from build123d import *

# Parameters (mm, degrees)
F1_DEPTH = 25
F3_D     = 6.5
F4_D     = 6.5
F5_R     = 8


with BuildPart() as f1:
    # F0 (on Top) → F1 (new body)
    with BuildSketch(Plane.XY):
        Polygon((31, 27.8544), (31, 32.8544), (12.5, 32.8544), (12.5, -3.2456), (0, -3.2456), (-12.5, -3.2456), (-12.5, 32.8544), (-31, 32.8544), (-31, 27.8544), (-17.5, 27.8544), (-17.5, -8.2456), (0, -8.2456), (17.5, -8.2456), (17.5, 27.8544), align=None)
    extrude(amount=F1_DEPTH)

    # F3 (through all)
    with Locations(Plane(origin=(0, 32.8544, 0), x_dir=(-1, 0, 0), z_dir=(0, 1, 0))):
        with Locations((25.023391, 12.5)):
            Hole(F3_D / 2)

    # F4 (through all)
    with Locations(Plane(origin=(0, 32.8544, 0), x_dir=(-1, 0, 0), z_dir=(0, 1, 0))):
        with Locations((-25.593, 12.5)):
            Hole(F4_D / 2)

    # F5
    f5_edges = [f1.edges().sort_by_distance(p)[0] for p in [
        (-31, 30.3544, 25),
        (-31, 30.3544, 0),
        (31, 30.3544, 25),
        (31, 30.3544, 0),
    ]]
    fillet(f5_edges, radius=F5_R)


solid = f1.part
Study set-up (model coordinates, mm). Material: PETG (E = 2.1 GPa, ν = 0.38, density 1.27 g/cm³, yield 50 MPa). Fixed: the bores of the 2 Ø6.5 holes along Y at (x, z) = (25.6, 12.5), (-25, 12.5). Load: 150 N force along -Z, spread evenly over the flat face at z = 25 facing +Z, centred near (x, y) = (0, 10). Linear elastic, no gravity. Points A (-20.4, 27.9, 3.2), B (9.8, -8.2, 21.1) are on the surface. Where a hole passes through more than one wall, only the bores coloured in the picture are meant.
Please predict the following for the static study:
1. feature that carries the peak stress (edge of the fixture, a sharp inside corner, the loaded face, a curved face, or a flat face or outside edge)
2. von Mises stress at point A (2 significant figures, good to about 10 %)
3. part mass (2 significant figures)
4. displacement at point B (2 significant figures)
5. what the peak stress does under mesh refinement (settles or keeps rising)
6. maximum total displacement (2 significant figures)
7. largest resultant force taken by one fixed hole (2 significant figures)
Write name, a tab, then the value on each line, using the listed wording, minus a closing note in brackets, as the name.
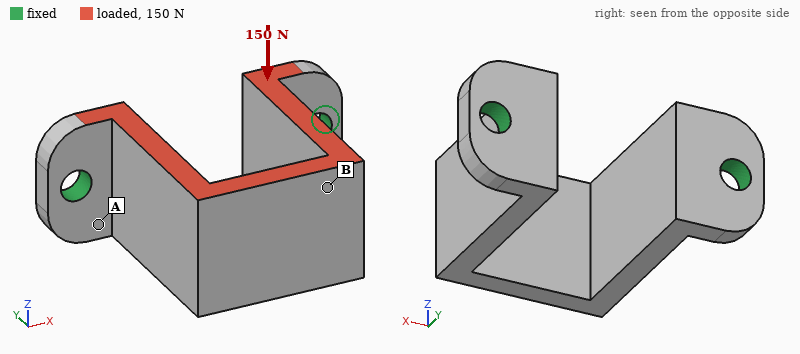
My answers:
feature that carries the peak stress	edge of the fixture
von Mises stress at point A	5.4 MPa
part mass	21 g
displacement at point B	0.60 mm
what the peak stress does under mesh refinement	keeps rising
maximum total displacement	0.62 mm
largest resultant force taken by one fixed hole	76 N
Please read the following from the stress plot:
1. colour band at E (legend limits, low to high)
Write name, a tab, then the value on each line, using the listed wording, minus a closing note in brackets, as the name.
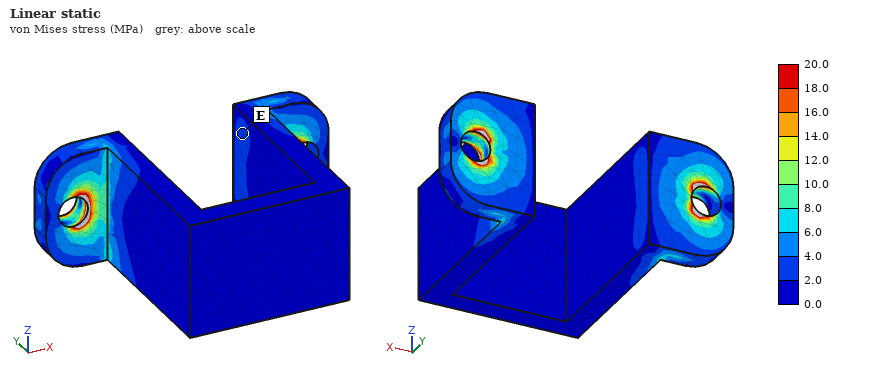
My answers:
colour band at E	2.0 to 4.0 MPa
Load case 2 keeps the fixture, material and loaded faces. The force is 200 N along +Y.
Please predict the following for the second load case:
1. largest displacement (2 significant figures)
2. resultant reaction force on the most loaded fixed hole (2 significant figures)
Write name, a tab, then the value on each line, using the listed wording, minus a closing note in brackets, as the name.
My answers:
largest displacement	0.51 mm
resultant reaction force on the most loaded fixed hole	100 N
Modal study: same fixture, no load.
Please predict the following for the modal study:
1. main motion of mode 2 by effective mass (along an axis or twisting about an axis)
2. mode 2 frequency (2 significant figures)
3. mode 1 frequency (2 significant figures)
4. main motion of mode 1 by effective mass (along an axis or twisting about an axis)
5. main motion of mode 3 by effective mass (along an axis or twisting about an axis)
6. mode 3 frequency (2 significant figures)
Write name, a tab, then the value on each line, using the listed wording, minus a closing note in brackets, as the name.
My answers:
main motion of mode 2 by effective mass	along X
mode 2 frequency	720 Hz
mode 1 frequency	650 Hz
main motion of mode 1 by effective mass	along Z
main motion of mode 3 by effective mass	twisting about Y
mode 3 frequency	1200 Hz
